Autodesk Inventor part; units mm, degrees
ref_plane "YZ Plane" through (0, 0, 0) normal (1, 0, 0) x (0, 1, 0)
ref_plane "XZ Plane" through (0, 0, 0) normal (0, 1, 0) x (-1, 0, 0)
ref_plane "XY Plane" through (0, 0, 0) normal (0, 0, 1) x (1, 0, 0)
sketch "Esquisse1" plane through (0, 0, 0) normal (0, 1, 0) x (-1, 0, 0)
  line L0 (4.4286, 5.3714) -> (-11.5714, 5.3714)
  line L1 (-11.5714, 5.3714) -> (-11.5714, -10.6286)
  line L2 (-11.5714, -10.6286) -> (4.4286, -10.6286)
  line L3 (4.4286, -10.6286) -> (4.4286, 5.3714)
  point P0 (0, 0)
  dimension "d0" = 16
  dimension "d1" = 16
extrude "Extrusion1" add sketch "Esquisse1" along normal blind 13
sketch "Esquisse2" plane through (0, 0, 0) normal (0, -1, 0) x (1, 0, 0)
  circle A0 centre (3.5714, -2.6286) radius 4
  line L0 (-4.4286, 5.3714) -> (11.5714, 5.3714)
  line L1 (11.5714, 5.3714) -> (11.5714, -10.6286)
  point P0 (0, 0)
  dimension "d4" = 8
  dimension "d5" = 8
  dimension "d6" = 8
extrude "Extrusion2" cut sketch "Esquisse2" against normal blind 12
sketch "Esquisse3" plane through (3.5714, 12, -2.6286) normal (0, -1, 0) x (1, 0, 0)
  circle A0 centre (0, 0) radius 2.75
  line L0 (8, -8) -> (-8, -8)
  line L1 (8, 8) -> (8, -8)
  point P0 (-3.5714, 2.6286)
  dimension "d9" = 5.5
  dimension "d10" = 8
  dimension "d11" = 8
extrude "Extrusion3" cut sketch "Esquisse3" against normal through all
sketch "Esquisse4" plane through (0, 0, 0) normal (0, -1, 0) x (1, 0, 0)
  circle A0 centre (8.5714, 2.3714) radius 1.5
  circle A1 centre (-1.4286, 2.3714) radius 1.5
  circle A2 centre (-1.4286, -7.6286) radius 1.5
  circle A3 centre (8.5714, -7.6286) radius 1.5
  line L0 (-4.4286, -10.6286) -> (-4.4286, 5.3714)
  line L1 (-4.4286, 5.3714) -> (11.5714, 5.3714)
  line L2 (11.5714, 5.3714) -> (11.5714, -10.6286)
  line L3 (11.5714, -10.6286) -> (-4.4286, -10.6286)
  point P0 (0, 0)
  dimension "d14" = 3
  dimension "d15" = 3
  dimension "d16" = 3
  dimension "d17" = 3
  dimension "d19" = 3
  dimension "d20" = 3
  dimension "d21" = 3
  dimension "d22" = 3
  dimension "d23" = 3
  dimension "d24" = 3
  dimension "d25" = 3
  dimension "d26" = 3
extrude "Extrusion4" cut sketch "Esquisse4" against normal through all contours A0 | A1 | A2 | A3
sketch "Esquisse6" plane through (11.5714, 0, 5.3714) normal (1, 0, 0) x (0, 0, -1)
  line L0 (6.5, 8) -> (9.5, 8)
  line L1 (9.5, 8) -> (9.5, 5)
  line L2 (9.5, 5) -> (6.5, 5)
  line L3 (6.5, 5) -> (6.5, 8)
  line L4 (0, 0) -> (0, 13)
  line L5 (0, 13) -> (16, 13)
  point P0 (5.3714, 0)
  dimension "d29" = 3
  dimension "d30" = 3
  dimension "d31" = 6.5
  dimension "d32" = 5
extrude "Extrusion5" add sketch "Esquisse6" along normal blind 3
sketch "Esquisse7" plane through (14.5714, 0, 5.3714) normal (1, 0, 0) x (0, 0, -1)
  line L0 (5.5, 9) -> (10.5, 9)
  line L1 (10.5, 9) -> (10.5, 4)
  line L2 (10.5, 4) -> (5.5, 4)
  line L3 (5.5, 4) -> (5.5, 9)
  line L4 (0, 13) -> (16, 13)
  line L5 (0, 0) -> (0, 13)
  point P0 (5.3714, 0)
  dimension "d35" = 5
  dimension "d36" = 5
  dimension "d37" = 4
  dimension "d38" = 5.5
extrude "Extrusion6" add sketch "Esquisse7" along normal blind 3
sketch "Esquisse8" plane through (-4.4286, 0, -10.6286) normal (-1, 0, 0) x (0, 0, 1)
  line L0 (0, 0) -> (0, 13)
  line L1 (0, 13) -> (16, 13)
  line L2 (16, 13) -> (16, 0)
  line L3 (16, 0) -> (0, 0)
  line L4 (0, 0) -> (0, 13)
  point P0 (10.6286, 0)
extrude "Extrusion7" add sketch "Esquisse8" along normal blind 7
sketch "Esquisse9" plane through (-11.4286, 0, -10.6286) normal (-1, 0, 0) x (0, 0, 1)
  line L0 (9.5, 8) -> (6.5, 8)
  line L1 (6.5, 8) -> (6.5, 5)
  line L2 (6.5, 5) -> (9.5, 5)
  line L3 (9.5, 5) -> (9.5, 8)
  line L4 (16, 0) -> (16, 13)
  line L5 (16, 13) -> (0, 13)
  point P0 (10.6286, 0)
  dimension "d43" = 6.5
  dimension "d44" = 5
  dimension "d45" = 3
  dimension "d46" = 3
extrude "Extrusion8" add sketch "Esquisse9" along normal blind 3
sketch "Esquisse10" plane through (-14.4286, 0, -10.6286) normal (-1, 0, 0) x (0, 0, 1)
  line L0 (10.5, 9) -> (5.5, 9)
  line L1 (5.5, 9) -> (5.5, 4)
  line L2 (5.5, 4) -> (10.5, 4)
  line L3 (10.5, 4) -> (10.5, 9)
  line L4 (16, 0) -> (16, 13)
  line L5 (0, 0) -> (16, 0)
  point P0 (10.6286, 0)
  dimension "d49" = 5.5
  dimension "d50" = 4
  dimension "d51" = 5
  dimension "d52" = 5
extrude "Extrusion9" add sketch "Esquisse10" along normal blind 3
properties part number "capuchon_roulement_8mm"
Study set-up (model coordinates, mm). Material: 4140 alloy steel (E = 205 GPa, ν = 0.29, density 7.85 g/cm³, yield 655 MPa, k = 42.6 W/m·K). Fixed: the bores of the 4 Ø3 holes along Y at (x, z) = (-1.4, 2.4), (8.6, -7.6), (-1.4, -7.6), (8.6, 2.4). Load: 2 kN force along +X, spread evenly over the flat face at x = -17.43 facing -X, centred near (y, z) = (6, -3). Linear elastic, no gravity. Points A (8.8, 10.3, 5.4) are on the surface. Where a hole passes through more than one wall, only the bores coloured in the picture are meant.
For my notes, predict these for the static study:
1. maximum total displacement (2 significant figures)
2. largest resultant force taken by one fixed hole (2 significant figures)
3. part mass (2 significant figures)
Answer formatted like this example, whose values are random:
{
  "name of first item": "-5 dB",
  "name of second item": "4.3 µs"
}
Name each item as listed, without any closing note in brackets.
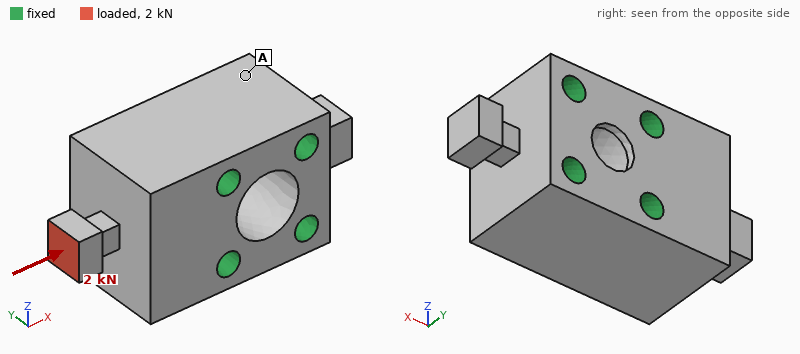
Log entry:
{
  "maximum total displacement": "7.4 µm",
  "largest resultant force taken by one fixed hole": "1.1 kN",
  "part mass": "31 g"
}
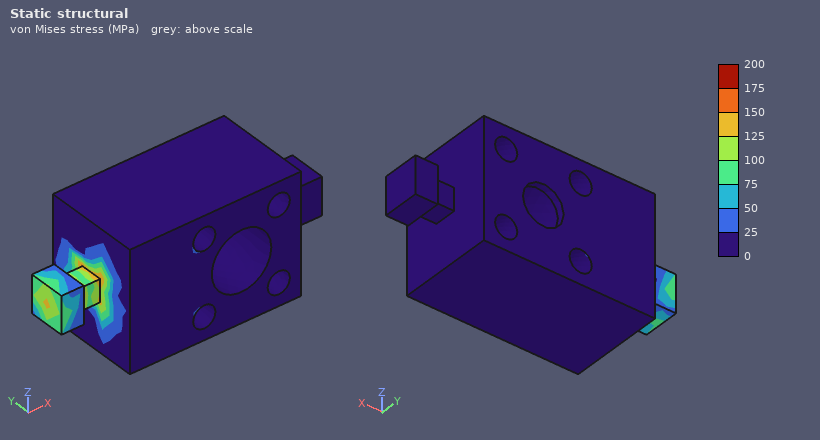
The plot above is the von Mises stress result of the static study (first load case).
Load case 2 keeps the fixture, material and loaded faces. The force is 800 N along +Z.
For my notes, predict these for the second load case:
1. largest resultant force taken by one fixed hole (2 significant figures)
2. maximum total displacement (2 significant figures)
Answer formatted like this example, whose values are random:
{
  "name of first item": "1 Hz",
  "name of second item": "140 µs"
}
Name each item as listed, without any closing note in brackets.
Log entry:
{
  "largest resultant force taken by one fixed hole": "1.1 kN",
  "maximum total displacement": "66 µm"
}
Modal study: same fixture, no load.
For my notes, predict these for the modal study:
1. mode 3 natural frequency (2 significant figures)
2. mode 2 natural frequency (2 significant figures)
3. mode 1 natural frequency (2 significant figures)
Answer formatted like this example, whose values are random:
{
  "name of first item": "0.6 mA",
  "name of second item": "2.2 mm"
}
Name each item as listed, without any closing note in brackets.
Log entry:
{
  "mode 3 natural frequency": "30 kHz",
  "mode 2 natural frequency": "30 kHz",
  "mode 1 natural frequency": "30 kHz"
}
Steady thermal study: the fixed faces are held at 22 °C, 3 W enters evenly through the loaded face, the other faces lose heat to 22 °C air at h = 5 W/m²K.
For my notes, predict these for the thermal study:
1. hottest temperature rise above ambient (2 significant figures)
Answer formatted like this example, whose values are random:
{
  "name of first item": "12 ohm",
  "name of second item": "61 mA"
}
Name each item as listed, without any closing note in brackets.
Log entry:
{
  "hottest temperature rise above ambient": "45 K"
}
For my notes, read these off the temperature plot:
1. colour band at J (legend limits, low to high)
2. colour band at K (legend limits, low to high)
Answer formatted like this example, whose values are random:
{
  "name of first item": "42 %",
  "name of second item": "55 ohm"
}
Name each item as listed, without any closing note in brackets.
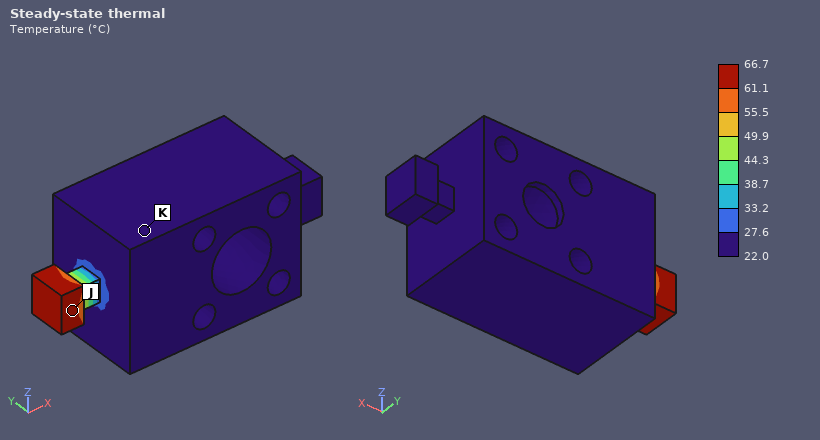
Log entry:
{
  "colour band at J": "61.1 to 66.7 °C",
  "colour band at K": "22.0 to 27.6 °C"
}
